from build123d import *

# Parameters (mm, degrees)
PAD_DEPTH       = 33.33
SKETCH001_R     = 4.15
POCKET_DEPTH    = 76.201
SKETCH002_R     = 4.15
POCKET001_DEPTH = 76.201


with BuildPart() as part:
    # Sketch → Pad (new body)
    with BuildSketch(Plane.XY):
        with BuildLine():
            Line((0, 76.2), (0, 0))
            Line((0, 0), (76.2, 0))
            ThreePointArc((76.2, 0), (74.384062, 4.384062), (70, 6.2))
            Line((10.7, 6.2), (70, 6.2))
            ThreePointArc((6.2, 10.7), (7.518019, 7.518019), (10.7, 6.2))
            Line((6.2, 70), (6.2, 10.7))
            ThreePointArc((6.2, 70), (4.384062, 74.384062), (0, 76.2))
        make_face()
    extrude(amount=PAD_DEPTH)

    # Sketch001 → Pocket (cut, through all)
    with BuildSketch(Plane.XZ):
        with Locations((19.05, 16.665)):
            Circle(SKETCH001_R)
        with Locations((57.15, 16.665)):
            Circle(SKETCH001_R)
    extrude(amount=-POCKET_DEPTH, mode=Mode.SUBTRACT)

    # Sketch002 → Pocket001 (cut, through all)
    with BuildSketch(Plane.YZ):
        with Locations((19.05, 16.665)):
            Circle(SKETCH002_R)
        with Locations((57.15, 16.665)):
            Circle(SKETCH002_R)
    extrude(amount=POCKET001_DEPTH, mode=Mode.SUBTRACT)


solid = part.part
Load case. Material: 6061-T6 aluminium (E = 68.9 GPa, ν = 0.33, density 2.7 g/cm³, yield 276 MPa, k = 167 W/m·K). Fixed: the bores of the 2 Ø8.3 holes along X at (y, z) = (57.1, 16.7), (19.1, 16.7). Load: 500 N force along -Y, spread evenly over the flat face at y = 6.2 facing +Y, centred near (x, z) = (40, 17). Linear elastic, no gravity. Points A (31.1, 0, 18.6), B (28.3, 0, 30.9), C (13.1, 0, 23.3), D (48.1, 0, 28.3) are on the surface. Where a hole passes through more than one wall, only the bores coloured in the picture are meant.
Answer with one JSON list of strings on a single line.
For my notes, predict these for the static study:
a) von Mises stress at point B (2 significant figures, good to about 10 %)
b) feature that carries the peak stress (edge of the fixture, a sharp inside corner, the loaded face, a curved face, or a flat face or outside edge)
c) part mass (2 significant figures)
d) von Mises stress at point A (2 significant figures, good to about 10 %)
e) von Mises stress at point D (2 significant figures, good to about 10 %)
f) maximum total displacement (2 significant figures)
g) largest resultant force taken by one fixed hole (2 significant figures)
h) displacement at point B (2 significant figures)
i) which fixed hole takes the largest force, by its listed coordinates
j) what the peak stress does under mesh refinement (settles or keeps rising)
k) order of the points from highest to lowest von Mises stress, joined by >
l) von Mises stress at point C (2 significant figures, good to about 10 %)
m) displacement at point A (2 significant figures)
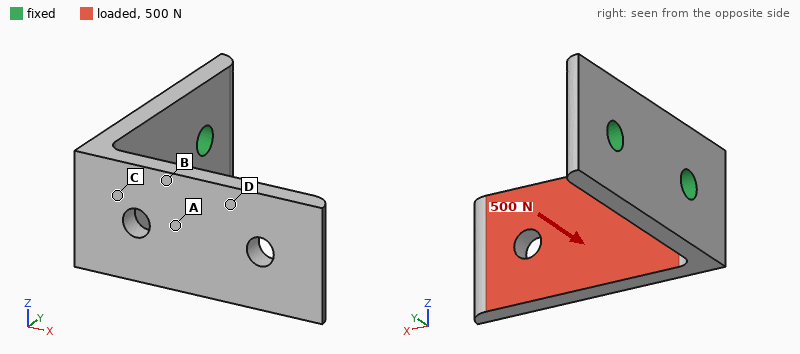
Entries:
["39 MPa", "edge of the fixture", "77 g", "26 MPa", "11 MPa", "0.82 mm", "470 N", "0.21 mm", "(19.1, 16.7)", "keeps rising", "C > B > A > D", "67 MPa", "0.24 mm"]
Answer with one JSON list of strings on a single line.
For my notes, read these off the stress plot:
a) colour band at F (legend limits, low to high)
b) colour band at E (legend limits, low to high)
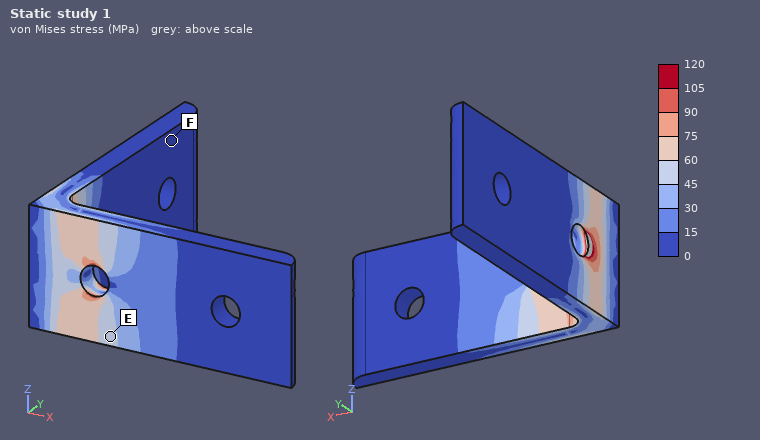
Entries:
["0 to 15 MPa", "45 to 60 MPa"]
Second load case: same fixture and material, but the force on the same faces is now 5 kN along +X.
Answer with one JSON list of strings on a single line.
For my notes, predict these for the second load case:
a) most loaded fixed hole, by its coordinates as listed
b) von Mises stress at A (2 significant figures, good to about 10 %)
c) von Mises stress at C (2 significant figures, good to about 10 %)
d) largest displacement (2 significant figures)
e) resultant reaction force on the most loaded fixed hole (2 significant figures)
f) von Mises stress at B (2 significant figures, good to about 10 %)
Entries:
["(19.1, 16.7)", "30 MPa", "38 MPa", "0.15 mm", "5.2 kN", "38 MPa"]
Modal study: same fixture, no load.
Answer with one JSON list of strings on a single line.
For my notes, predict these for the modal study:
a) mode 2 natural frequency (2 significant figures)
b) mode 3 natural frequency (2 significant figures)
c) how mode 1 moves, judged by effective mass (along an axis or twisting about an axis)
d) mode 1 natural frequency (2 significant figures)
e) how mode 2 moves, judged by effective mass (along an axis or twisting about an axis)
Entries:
["1500 Hz", "4000 Hz", "along Y", "800 Hz", "along Z"]
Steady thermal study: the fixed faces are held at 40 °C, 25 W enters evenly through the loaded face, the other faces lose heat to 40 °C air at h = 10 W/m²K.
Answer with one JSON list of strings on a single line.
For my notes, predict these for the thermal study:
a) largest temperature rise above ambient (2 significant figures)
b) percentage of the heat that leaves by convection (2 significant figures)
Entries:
["36 K", "4.8 %"]
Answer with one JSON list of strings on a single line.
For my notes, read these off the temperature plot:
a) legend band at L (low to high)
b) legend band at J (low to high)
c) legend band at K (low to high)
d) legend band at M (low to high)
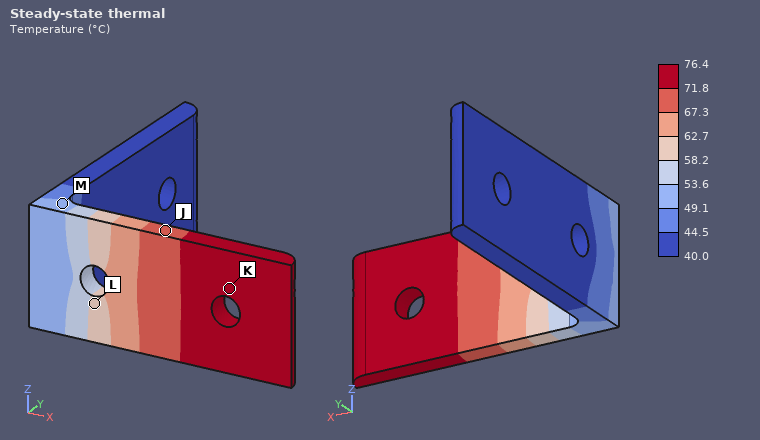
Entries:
["58.2 to 62.7 °C", "67.3 to 71.8 °C", "71.8 to 76.4 °C", "49.1 to 53.6 °C"]
